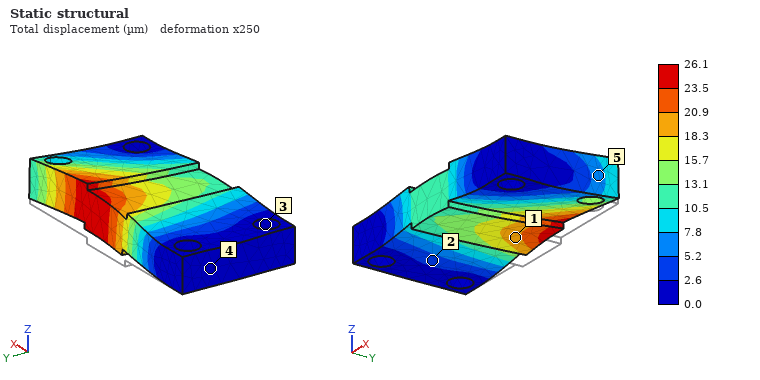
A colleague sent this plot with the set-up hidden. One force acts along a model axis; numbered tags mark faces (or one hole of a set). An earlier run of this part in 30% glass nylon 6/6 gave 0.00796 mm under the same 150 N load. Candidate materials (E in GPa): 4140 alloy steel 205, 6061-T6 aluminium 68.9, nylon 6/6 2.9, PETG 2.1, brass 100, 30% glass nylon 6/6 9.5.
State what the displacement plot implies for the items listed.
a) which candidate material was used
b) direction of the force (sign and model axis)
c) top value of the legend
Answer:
nylon 6/6
+Z
26.1 µm
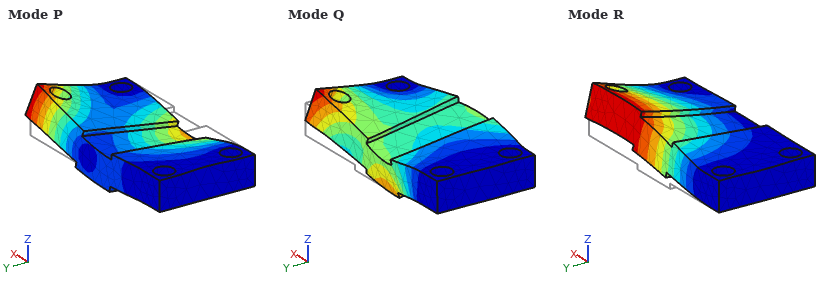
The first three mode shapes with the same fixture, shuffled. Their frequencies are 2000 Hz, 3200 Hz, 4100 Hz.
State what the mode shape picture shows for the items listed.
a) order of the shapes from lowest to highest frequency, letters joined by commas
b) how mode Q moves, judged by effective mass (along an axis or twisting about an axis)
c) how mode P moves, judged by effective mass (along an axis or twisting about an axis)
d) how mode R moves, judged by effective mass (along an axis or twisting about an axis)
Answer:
R, P, Q
along Y
along Z
along Z
